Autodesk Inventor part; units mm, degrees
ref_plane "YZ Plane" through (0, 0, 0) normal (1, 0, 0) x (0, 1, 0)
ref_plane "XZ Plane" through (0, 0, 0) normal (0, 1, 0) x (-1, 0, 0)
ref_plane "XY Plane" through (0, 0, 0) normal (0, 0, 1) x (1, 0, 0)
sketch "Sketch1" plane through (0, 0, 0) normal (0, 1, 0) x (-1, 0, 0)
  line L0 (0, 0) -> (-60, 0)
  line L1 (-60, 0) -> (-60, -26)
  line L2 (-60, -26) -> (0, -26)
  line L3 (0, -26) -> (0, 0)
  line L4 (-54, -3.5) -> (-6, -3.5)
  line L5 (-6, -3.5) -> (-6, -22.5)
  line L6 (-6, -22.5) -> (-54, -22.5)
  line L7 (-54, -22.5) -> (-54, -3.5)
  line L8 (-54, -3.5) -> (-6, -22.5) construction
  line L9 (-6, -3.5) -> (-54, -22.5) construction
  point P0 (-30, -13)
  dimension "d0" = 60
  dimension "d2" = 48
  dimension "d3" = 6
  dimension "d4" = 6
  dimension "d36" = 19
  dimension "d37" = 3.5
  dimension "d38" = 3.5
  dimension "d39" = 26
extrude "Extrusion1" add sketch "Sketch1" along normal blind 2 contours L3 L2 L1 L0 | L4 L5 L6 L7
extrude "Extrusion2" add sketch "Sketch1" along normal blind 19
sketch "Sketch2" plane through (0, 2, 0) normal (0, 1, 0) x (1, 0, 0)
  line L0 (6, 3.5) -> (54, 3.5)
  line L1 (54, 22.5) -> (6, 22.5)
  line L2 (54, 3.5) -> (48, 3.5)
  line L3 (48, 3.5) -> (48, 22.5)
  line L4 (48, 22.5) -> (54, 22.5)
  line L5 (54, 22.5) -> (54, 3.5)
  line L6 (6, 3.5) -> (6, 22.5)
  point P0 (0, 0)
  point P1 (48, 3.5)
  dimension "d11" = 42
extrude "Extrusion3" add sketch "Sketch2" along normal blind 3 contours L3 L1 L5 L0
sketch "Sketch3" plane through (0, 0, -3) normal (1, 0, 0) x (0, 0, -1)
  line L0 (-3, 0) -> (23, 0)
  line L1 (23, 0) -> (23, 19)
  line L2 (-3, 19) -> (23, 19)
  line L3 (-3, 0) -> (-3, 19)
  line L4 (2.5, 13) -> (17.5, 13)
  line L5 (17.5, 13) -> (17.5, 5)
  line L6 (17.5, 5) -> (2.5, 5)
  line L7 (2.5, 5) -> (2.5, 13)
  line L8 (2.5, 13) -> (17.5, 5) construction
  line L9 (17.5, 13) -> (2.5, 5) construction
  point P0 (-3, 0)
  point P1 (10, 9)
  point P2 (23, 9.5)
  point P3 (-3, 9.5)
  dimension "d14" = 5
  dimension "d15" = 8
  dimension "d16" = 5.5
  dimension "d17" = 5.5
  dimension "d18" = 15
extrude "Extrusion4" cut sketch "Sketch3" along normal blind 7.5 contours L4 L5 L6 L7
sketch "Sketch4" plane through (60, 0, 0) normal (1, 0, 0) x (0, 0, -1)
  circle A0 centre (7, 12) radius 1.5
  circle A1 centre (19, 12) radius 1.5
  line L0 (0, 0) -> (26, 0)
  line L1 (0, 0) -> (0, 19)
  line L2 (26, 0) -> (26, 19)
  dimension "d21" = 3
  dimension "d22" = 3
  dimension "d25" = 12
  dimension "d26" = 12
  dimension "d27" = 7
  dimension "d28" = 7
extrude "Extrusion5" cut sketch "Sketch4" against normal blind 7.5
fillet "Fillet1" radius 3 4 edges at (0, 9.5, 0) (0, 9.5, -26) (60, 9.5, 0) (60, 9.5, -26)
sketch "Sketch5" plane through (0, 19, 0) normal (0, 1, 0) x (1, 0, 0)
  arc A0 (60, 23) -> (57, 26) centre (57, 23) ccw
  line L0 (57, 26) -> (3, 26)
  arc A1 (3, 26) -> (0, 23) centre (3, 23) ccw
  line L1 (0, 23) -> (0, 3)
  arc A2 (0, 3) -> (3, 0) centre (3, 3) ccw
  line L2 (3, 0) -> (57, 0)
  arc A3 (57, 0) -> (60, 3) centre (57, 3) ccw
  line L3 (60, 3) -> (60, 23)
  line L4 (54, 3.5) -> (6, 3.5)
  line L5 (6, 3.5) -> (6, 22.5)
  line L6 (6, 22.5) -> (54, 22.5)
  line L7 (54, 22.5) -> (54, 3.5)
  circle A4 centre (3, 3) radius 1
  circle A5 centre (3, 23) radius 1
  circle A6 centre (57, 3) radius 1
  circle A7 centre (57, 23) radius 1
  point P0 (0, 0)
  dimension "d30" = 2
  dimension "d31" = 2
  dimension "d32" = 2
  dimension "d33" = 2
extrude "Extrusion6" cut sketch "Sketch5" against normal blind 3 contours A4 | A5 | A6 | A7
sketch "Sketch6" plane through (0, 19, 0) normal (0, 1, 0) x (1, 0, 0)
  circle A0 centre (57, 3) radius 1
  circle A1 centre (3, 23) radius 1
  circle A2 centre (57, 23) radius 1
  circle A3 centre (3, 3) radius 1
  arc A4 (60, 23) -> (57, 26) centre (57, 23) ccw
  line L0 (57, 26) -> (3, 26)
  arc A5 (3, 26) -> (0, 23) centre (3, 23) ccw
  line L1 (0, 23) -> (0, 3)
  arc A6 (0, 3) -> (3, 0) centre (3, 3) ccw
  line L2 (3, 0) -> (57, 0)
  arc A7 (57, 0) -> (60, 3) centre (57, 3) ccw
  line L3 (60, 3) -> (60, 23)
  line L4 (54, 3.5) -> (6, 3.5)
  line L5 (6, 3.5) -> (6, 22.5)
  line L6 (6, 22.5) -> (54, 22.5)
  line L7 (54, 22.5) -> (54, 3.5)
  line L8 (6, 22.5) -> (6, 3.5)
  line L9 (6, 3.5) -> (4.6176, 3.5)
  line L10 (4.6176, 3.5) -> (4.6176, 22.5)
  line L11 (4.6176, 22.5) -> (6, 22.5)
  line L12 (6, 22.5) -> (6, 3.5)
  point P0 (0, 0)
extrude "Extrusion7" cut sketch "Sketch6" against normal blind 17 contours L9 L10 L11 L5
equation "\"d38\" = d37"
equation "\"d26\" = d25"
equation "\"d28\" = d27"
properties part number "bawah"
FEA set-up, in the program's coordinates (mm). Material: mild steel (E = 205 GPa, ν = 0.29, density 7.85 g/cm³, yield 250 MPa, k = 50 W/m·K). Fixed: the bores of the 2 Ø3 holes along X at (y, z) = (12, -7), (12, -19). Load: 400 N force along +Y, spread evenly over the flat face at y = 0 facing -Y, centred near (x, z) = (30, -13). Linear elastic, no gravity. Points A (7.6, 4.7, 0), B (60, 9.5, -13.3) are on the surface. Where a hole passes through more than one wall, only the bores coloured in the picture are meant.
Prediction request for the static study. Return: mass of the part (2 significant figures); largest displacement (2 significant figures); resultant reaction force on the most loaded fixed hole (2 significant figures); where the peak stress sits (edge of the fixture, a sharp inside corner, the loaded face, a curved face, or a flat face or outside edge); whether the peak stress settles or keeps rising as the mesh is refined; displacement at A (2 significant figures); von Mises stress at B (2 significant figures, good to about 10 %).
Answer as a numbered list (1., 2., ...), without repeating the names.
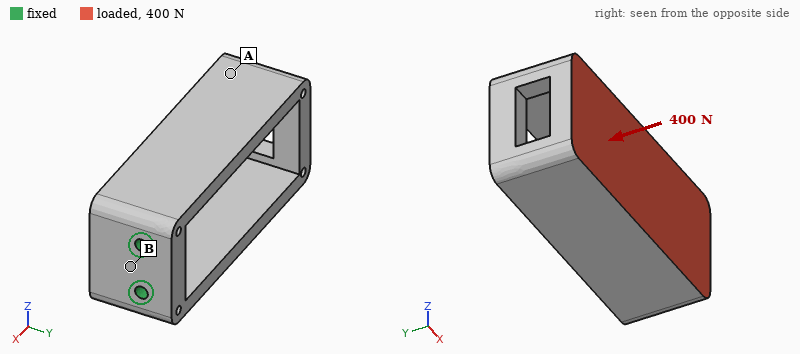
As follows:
1. 100 g
2. 31 µm
3. 200 N
4. edge of the fixture
5. keeps rising
6. 26 µm
7. 19 MPa
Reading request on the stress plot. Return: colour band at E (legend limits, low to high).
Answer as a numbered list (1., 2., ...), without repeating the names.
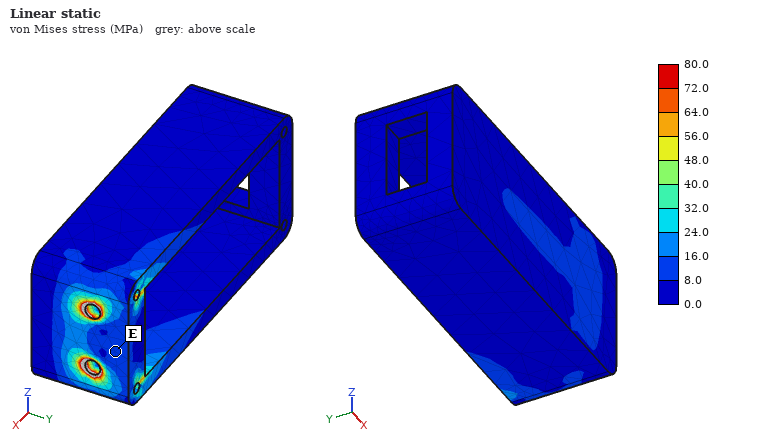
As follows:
1. 8.0 to 16.0 MPa
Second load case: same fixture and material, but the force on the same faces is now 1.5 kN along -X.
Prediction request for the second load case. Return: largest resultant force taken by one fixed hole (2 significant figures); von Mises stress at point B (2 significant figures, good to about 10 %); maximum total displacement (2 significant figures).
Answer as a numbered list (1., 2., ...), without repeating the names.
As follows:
1. 750 N
2. 36 MPa
3. 45 µm
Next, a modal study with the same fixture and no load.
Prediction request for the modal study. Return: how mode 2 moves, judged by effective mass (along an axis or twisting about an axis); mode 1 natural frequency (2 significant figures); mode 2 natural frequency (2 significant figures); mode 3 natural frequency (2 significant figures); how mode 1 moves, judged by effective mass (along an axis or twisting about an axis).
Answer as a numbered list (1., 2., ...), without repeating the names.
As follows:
1. along Y
2. 2000 Hz
3. 2200 Hz
4. 6600 Hz
5. along Z
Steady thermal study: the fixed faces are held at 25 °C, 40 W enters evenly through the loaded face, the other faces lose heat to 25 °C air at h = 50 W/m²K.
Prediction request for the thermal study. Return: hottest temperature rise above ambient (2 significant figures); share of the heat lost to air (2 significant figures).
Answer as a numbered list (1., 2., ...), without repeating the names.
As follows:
1. 79 K
2. 40 %
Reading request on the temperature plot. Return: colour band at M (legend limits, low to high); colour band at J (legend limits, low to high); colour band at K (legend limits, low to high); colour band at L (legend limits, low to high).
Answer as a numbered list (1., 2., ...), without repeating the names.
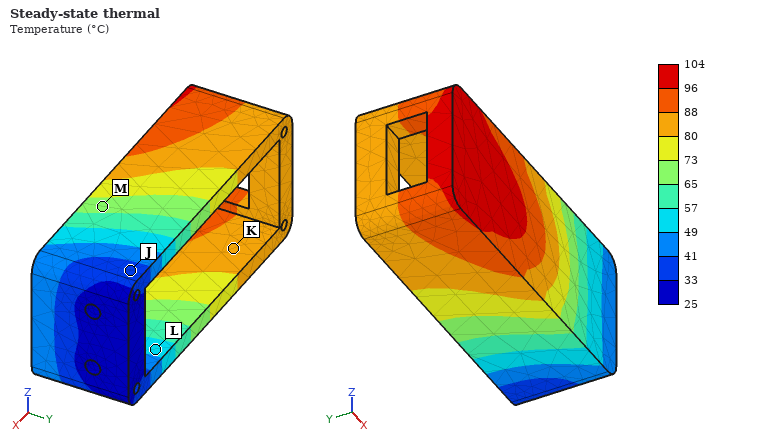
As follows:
1. 65 to 73 °C
2. 33 to 41 °C
3. 80 to 88 °C
4. 49 to 57 °C
